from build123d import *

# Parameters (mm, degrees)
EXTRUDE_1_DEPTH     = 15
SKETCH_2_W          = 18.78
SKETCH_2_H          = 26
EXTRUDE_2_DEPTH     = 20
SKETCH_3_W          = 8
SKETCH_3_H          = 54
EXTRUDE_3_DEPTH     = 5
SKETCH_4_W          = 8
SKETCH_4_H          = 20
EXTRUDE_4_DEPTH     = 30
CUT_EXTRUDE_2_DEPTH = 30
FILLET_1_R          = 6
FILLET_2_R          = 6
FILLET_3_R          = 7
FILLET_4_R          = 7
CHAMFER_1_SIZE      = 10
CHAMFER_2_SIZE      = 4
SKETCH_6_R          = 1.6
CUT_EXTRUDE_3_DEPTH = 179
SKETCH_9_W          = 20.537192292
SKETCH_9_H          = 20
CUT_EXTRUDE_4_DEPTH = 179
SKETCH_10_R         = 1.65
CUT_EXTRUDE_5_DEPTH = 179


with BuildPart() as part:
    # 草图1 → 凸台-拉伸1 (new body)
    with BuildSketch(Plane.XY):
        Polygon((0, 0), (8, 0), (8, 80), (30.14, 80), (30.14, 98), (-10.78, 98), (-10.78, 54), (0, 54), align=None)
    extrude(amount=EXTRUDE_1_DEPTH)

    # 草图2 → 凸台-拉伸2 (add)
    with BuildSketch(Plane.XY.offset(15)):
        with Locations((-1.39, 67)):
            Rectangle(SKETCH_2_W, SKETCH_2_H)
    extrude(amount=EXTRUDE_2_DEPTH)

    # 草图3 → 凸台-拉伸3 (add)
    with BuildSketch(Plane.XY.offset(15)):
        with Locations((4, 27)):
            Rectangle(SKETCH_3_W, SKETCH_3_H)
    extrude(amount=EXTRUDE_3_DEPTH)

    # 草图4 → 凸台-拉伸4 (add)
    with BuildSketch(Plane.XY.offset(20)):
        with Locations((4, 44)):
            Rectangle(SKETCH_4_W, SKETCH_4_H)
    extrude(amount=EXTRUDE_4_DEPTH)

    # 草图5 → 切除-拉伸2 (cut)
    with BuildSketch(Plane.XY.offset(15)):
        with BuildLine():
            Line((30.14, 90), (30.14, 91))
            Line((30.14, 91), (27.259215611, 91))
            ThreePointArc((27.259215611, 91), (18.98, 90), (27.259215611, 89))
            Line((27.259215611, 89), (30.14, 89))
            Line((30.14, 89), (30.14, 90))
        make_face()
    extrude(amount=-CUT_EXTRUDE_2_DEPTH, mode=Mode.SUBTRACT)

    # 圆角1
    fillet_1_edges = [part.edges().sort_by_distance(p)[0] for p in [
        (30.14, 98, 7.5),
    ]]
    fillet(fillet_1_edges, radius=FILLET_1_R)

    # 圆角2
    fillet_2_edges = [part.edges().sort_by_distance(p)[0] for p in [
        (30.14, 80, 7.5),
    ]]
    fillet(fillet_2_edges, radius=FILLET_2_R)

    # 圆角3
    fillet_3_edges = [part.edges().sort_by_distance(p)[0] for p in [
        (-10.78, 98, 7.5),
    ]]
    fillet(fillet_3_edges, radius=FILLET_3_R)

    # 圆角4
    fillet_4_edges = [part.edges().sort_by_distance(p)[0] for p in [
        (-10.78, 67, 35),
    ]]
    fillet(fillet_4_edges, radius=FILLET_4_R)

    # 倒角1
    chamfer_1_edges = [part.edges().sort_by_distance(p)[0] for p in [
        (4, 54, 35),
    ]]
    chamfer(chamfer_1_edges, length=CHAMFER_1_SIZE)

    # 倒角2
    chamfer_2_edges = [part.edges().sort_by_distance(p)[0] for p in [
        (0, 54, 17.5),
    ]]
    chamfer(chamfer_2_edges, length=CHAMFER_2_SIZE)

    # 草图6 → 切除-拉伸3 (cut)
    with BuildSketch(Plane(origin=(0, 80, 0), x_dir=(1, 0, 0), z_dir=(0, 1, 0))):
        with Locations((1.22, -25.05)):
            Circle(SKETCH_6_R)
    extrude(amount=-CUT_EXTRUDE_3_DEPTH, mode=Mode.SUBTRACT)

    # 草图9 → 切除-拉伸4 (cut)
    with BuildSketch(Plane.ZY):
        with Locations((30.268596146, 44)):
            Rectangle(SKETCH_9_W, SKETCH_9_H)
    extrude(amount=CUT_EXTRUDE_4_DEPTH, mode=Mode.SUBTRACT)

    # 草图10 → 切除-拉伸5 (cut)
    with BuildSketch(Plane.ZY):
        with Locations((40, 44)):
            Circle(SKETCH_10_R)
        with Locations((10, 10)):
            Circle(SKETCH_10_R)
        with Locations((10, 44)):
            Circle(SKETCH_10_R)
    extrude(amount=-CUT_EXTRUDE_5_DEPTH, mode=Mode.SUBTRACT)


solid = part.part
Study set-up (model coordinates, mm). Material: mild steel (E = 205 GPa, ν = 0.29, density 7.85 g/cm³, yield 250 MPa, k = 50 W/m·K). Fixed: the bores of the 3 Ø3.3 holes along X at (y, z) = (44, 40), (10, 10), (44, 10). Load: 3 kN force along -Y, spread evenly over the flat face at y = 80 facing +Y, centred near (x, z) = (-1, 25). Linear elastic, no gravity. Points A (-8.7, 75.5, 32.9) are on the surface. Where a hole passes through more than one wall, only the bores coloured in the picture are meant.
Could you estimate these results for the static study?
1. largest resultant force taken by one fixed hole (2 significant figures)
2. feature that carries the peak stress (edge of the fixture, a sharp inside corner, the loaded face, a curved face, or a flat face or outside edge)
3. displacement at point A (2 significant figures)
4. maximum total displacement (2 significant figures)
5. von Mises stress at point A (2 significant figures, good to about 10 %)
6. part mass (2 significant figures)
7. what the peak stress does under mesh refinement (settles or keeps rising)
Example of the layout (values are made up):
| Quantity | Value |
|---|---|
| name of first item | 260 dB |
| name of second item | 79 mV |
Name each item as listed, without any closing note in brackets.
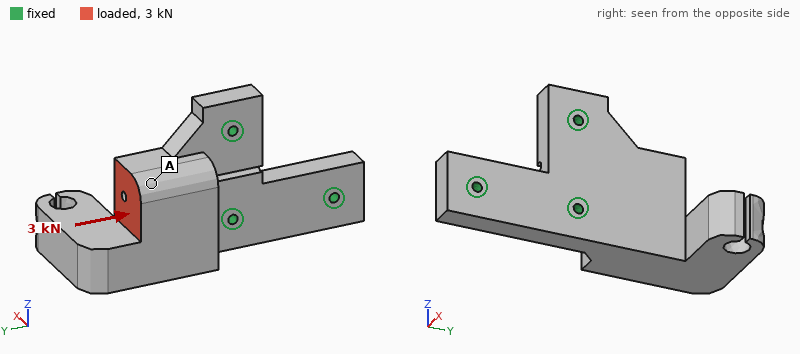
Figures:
| Quantity | Value |
|---|---|
| largest resultant force taken by one fixed hole | 1.5 kN |
| feature that carries the peak stress | edge of the fixture |
| displacement at point A | 19 µm |
| maximum total displacement | 33 µm |
| von Mises stress at point A | 8.7 MPa |
| part mass | 310 g |
| what the peak stress does under mesh refinement | keeps rising |
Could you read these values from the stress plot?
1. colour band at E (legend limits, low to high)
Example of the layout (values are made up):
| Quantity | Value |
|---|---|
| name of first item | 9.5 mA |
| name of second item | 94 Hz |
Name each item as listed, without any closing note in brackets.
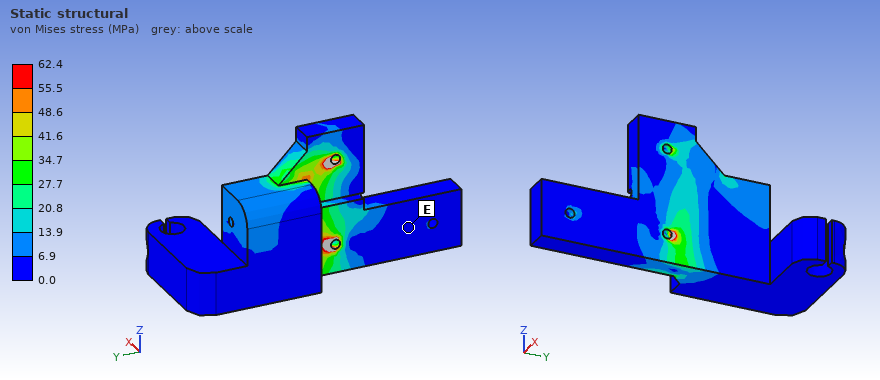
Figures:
| Quantity | Value |
|---|---|
| colour band at E | 0.0 to 6.9 MPa |
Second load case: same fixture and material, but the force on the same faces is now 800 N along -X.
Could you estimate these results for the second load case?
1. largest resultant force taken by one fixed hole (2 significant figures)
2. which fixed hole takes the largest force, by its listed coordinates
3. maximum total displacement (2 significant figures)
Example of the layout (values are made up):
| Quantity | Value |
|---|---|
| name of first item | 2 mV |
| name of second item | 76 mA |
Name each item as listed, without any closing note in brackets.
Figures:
| Quantity | Value |
|---|---|
| largest resultant force taken by one fixed hole | 540 N |
| which fixed hole takes the largest force, by its listed coordinates | (44, 10) |
| maximum total displacement | 54 µm |
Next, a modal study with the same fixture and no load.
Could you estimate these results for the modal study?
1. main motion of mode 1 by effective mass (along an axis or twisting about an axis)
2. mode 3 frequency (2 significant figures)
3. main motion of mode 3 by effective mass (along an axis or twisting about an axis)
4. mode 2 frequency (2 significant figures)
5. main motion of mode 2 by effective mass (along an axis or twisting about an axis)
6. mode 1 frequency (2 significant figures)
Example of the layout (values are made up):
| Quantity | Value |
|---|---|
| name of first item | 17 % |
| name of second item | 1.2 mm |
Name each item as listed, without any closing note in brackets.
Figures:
| Quantity | Value |
|---|---|
| main motion of mode 1 by effective mass | along X |
| mode 3 frequency | 7800 Hz |
| main motion of mode 3 by effective mass | along Z |
| mode 2 frequency | 5200 Hz |
| main motion of mode 2 by effective mass | along Z |
| mode 1 frequency | 1700 Hz |
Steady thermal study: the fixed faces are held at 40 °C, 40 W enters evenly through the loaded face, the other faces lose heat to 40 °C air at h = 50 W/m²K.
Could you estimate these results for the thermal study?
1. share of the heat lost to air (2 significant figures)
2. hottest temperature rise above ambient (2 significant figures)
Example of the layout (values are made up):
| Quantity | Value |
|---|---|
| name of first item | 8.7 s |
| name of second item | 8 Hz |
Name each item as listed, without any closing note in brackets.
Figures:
| Quantity | Value |
|---|---|
| share of the heat lost to air | 32 % |
| hottest temperature rise above ambient | 65 K |
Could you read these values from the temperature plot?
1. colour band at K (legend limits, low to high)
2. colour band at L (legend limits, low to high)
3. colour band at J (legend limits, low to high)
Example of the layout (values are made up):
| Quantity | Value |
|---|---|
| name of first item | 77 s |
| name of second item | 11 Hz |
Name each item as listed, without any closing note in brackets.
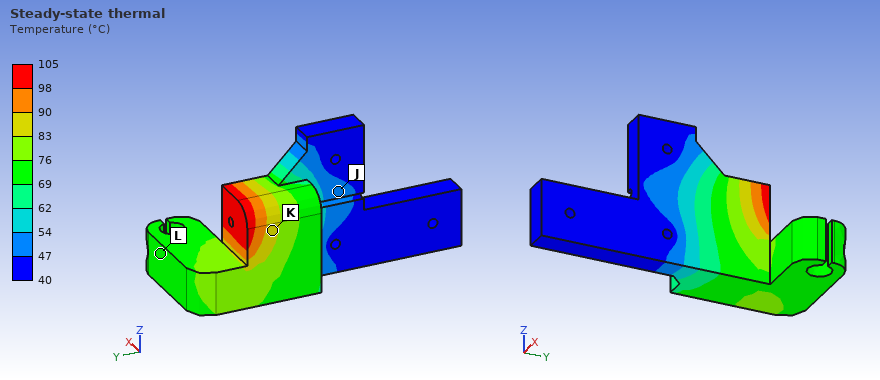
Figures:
| Quantity | Value |
|---|---|
| colour band at K | 83 to 90 °C |
| colour band at L | 69 to 76 °C |
| colour band at J | 47 to 54 °C |
